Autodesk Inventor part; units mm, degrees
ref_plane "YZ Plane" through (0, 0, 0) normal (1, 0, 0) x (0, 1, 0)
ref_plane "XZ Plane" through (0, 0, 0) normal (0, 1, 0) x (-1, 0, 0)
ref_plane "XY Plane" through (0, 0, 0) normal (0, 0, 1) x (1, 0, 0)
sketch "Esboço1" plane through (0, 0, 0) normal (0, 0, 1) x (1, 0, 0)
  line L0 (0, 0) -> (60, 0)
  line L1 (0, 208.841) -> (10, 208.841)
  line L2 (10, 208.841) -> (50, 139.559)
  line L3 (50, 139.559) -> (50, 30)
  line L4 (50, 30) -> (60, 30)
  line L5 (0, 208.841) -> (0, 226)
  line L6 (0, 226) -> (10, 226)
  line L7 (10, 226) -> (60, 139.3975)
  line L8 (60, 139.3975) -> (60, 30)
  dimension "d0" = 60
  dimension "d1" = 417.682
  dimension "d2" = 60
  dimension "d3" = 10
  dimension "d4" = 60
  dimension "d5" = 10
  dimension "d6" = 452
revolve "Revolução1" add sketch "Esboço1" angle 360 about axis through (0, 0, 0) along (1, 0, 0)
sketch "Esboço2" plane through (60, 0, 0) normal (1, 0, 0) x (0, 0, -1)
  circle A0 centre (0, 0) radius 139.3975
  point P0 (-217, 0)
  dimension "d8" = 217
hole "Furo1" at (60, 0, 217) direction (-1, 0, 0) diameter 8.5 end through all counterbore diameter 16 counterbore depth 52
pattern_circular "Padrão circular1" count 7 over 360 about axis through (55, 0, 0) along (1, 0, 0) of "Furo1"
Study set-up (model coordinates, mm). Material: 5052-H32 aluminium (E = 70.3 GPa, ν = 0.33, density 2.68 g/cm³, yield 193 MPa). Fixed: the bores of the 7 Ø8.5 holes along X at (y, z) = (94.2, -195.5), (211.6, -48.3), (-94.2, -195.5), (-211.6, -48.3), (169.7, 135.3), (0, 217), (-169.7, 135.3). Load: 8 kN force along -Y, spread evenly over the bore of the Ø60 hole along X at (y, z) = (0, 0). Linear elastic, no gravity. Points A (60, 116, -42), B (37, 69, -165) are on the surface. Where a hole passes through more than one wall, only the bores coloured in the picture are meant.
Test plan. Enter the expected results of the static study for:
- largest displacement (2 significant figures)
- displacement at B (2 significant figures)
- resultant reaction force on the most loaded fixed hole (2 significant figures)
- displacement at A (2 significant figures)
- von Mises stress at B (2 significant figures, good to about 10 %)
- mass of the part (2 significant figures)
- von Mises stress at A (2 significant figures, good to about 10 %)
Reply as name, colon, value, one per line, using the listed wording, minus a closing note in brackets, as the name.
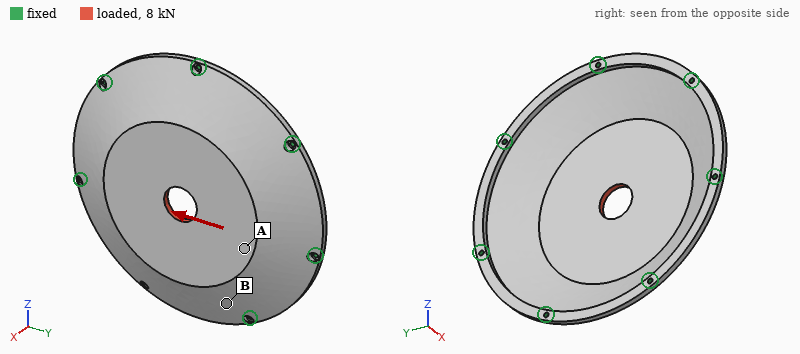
largest displacement: 21 µm
displacement at B: 6.0 µm
resultant reaction force on the most loaded fixed hole: 1.5 kN
displacement at A: 19 µm
von Mises stress at B: 1.7 MPa
mass of the part: 4.5 kg
von Mises stress at A: 3.5 MPa
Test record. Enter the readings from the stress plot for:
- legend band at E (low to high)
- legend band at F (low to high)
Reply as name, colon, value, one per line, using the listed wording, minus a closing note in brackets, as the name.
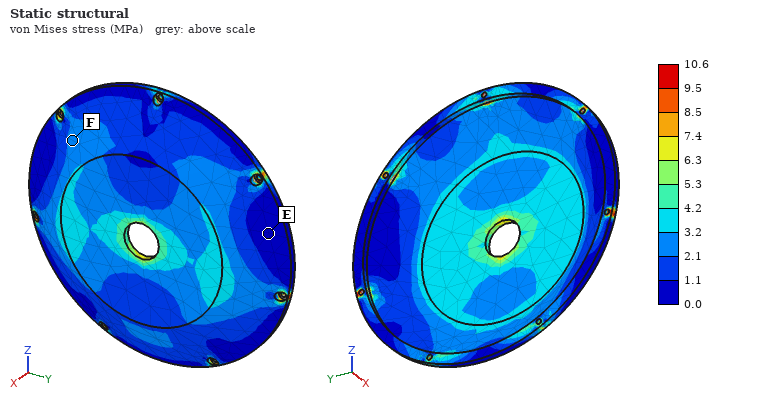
legend band at E: 0.0 to 1.1 MPa
legend band at F: 2.1 to 3.2 MPa
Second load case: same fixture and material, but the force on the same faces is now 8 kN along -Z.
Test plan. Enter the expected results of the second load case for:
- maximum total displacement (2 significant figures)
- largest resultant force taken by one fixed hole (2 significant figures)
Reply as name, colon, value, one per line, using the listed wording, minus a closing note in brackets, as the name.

maximum total displacement: 21 µm
largest resultant force taken by one fixed hole: 1.4 kN
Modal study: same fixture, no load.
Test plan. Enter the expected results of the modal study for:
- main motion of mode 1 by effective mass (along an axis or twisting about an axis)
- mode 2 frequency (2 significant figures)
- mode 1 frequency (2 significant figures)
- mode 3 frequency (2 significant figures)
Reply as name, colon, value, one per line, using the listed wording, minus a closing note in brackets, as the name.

main motion of mode 1 by effective mass: along X
mode 2 frequency: 1600 Hz
mode 1 frequency: 890 Hz
mode 3 frequency: 1600 Hz
